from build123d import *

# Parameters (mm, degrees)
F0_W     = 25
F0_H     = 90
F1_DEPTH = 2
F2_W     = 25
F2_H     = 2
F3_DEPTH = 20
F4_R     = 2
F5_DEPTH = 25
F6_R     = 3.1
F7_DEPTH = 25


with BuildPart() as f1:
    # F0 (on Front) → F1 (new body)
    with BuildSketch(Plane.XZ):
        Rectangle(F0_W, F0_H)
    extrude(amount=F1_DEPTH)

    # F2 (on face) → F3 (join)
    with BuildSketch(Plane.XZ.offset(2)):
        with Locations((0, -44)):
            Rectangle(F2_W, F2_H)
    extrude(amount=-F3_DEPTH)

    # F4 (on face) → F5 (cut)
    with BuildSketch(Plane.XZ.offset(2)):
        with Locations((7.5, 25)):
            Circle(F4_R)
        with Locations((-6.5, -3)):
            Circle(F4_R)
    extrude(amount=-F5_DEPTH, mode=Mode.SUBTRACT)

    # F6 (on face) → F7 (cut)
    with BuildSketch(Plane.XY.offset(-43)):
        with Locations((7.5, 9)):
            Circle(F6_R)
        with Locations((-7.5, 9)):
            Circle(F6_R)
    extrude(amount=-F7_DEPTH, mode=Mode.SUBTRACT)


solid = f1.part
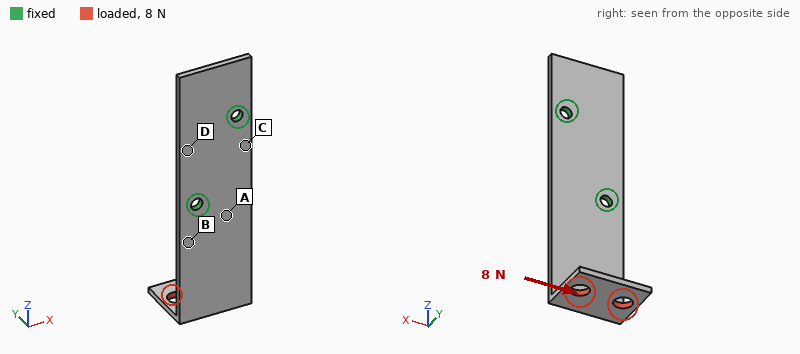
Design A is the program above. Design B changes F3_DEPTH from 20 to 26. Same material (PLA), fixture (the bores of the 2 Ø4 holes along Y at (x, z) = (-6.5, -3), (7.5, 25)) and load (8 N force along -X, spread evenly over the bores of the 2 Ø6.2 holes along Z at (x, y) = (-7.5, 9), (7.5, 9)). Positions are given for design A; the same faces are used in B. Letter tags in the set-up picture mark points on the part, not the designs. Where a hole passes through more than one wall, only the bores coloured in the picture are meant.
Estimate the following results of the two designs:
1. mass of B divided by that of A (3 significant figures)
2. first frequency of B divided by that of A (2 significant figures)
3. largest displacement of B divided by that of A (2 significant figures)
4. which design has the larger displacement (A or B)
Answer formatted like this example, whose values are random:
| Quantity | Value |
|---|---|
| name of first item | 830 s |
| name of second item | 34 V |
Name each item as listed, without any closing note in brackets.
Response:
| Quantity | Value |
|---|---|
| mass of B divided by that of A | 1.06 |
| first frequency of B divided by that of A | 0.86 |
| largest displacement of B divided by that of A | 1.2 |
| which design has the larger displacement | B |
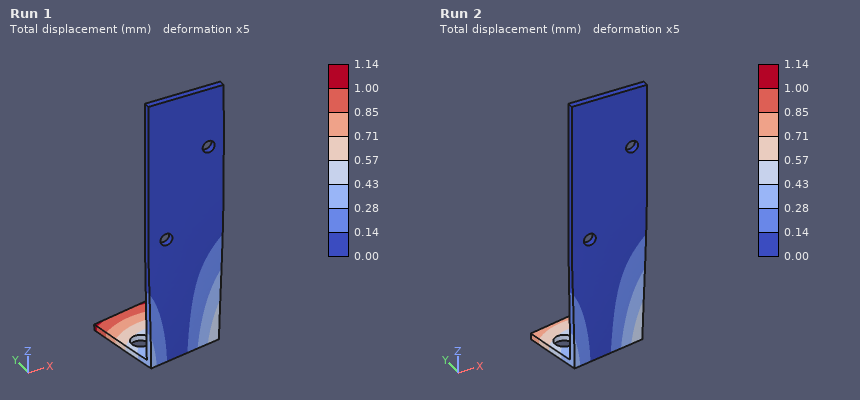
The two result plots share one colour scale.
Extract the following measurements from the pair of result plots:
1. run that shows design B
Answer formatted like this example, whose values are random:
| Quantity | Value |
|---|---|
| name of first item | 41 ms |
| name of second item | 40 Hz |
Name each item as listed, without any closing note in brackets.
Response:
| Quantity | Value |
|---|---|
| run that shows design B | Run 1 |
